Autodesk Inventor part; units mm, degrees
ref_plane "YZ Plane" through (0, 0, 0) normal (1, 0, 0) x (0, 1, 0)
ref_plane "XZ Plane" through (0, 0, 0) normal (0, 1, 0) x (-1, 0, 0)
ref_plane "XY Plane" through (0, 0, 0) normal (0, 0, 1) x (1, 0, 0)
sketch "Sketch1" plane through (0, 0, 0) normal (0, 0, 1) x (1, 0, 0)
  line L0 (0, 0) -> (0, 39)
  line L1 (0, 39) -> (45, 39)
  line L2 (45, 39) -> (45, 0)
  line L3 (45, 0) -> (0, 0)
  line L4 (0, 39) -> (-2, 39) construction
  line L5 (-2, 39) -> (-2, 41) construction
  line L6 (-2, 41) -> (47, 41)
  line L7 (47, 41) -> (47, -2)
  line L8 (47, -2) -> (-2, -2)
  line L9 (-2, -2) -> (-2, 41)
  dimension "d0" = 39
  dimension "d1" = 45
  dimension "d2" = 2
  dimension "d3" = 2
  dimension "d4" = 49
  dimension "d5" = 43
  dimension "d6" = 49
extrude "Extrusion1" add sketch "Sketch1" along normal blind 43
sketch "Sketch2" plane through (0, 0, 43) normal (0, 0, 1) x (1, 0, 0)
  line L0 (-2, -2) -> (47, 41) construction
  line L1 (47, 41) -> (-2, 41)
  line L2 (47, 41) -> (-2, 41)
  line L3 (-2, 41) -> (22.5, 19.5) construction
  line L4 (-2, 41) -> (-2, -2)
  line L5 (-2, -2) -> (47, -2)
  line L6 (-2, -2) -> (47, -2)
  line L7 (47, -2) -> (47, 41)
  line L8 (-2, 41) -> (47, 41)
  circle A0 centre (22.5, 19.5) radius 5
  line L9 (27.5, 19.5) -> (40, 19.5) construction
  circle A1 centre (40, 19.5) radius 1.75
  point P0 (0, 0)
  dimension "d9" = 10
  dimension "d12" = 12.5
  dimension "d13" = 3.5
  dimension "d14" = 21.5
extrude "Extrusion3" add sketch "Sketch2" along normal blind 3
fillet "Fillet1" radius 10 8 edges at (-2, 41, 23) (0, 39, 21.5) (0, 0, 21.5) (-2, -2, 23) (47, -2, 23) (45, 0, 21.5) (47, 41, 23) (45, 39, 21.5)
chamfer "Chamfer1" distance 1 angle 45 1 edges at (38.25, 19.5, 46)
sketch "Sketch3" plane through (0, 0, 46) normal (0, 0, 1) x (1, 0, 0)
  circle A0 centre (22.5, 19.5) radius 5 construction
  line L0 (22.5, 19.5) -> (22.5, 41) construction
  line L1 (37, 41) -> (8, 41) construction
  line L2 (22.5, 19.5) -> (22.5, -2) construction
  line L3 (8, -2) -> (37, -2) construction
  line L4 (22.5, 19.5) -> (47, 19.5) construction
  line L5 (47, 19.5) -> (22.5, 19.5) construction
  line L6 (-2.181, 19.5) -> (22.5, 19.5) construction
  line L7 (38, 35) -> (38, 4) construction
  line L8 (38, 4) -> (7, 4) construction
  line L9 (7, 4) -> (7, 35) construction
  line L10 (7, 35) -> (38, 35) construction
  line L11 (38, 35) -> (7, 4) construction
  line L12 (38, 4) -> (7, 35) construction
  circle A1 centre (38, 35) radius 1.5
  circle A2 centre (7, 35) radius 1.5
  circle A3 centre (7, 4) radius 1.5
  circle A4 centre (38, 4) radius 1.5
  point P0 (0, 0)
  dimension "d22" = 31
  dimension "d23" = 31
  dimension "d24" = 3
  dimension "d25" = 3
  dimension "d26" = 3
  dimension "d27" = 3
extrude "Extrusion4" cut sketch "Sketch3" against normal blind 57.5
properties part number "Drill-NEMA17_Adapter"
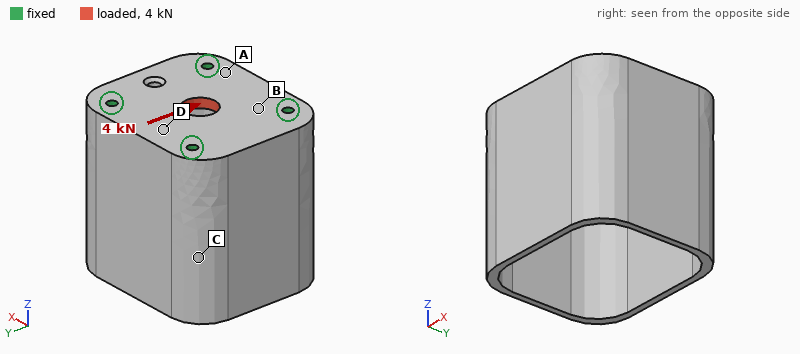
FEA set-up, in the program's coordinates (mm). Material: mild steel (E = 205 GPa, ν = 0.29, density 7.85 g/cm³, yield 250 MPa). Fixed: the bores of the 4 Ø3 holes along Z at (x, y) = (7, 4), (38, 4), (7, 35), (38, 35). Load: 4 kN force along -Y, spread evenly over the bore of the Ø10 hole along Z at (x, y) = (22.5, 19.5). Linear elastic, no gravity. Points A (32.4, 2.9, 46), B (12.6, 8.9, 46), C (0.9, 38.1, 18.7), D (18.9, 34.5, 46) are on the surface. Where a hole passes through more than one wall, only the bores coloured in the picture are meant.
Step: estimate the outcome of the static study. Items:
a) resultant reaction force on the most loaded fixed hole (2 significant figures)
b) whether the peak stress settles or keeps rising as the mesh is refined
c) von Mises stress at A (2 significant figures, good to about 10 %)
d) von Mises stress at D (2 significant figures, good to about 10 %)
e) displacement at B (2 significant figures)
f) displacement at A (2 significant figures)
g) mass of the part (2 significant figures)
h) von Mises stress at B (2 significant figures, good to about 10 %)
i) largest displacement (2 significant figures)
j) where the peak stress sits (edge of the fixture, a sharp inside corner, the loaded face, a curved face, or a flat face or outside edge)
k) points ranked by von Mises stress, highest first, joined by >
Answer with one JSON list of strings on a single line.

["1.1 kN", "keeps rising", "24 MPa", "16 MPa", "1.6 µm", "1.4 µm", "160 g", "34 MPa", "4.0 µm", "edge of the fixture", "B > A > D > C"]
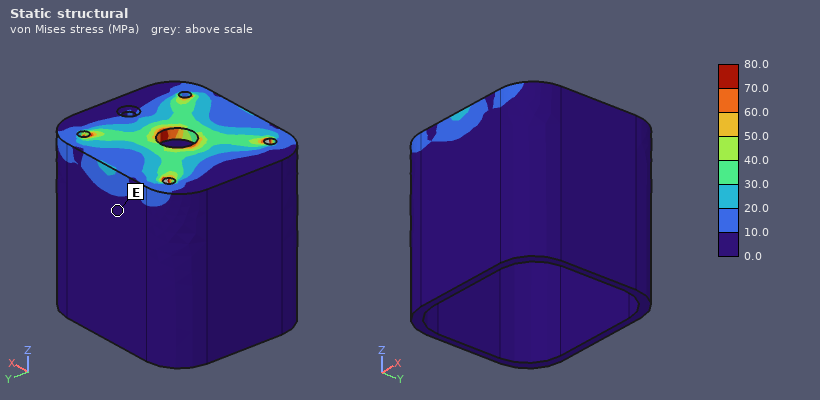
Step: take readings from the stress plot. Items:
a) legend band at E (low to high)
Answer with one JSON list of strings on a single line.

["0.0 to 10.0 MPa"]
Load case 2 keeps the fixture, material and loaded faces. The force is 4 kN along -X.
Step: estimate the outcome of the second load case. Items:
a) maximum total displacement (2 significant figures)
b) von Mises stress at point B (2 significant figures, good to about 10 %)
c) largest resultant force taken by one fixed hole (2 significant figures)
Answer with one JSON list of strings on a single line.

["3.8 µm", "32 MPa", "1.0 kN"]
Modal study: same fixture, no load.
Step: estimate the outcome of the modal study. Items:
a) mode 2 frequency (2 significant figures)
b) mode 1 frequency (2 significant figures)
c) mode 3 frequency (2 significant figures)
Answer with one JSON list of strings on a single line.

["5100 Hz", "3400 Hz", "5300 Hz"]
